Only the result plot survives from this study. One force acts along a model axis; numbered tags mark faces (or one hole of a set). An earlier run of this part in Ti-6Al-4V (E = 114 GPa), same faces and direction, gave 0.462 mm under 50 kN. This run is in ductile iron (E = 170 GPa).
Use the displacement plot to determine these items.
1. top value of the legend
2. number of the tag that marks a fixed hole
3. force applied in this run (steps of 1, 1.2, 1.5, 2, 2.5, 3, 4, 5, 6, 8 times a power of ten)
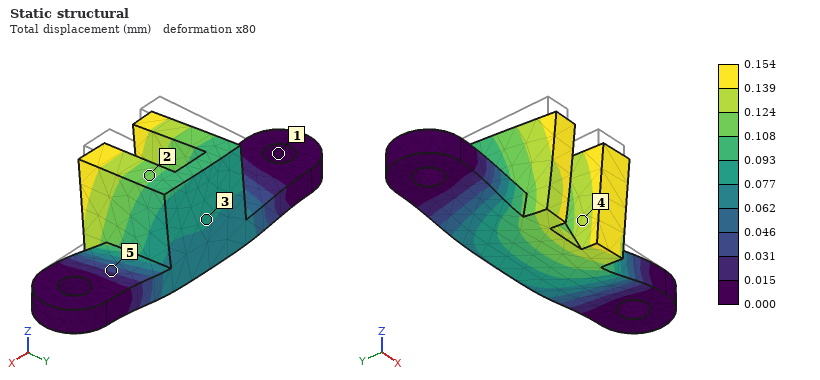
0.154 mm
1
25 kN
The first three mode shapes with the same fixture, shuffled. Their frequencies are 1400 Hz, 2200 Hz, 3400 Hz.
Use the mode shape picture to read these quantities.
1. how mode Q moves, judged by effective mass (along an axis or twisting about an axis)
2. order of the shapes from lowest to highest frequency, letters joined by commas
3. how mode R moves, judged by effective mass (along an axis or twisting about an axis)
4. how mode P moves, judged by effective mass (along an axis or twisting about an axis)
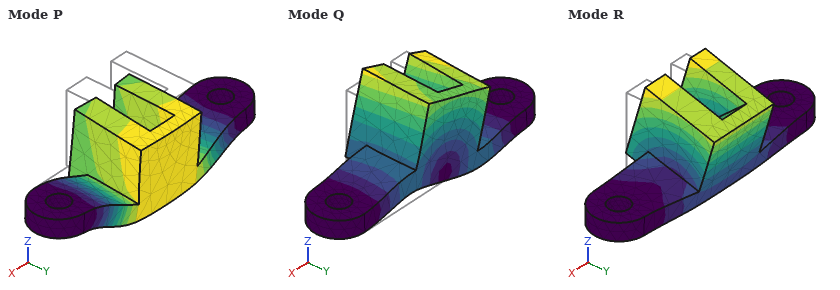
along X
R, P, Q
along Y
along Z
